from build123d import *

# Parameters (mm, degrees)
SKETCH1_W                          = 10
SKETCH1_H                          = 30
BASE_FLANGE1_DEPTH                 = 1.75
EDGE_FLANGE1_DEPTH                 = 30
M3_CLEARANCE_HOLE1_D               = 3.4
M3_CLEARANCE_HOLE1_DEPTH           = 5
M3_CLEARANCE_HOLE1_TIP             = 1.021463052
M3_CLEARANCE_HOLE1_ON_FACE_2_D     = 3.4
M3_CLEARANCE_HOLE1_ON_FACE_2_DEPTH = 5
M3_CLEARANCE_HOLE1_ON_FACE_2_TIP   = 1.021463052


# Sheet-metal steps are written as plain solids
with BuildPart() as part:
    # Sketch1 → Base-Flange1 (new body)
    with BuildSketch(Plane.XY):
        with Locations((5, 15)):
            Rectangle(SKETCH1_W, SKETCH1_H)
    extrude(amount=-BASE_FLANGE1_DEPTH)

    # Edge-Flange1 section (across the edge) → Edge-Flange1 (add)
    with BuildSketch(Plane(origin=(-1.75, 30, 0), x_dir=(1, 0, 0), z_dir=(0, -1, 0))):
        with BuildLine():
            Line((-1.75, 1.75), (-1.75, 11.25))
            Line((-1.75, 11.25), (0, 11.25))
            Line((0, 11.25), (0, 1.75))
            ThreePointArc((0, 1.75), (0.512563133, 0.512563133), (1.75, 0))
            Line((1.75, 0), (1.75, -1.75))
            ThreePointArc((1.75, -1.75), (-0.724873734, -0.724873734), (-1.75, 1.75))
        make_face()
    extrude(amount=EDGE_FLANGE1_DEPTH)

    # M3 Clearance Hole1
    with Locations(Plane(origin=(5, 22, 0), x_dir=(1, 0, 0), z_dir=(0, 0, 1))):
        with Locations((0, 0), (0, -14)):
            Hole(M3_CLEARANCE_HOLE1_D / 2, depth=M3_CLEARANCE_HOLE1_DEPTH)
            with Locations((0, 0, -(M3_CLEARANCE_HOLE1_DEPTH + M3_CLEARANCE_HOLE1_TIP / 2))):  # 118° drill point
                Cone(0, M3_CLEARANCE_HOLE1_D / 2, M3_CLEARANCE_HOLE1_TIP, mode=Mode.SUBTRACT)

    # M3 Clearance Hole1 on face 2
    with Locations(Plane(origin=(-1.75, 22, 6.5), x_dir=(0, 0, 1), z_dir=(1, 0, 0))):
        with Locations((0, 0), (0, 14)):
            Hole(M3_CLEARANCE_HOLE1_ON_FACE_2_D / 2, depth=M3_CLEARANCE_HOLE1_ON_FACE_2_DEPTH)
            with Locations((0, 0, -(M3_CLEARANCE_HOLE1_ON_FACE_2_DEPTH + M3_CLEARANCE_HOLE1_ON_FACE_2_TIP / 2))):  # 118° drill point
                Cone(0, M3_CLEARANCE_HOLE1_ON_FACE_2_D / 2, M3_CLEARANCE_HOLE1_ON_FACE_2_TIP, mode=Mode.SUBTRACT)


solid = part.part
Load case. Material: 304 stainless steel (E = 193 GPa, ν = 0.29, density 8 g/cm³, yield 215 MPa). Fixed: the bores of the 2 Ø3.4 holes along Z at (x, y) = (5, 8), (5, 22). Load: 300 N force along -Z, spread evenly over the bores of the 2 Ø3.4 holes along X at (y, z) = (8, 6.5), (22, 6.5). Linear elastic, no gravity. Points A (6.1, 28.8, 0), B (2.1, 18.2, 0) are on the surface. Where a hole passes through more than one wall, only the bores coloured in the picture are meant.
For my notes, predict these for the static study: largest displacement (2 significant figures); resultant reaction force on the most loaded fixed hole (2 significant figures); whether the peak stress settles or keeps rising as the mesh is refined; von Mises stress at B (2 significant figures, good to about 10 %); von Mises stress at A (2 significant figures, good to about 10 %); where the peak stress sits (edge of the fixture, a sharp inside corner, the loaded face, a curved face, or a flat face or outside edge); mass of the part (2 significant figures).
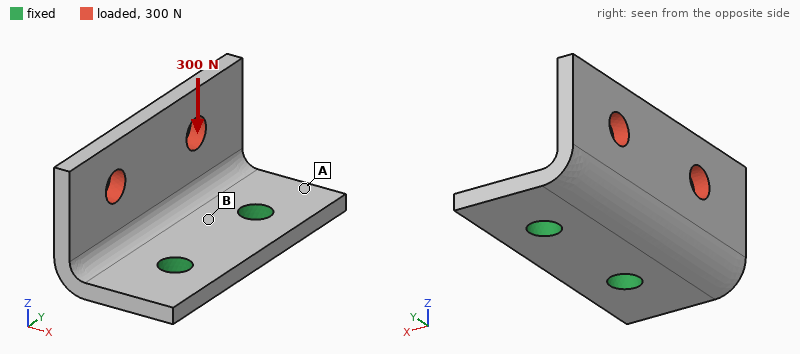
40 µm
150 N
keeps rising
76 MPa
29 MPa
edge of the fixture
9.4 g
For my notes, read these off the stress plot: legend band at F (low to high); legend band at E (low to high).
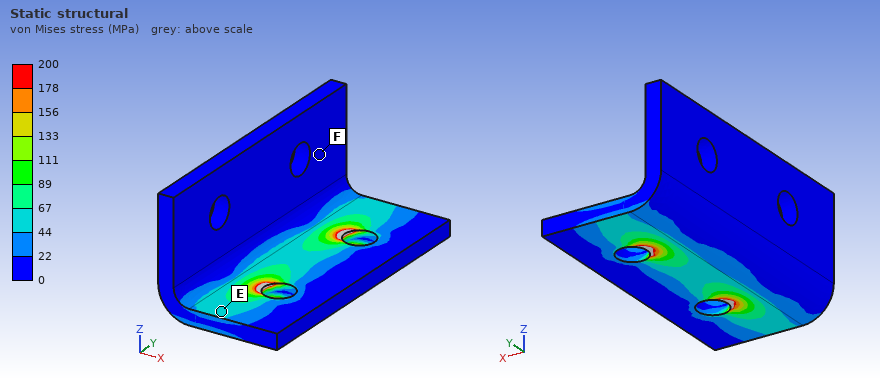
0 to 22 MPa
44 to 67 MPa
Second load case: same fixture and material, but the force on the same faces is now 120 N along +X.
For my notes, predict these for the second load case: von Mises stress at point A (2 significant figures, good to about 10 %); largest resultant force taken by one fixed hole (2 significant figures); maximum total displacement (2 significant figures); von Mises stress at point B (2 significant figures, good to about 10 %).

15 MPa
61 N
38 µm
51 MPa
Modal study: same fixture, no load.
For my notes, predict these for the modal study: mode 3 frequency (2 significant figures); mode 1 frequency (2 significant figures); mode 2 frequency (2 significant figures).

14 kHz
5200 Hz
7700 Hz
